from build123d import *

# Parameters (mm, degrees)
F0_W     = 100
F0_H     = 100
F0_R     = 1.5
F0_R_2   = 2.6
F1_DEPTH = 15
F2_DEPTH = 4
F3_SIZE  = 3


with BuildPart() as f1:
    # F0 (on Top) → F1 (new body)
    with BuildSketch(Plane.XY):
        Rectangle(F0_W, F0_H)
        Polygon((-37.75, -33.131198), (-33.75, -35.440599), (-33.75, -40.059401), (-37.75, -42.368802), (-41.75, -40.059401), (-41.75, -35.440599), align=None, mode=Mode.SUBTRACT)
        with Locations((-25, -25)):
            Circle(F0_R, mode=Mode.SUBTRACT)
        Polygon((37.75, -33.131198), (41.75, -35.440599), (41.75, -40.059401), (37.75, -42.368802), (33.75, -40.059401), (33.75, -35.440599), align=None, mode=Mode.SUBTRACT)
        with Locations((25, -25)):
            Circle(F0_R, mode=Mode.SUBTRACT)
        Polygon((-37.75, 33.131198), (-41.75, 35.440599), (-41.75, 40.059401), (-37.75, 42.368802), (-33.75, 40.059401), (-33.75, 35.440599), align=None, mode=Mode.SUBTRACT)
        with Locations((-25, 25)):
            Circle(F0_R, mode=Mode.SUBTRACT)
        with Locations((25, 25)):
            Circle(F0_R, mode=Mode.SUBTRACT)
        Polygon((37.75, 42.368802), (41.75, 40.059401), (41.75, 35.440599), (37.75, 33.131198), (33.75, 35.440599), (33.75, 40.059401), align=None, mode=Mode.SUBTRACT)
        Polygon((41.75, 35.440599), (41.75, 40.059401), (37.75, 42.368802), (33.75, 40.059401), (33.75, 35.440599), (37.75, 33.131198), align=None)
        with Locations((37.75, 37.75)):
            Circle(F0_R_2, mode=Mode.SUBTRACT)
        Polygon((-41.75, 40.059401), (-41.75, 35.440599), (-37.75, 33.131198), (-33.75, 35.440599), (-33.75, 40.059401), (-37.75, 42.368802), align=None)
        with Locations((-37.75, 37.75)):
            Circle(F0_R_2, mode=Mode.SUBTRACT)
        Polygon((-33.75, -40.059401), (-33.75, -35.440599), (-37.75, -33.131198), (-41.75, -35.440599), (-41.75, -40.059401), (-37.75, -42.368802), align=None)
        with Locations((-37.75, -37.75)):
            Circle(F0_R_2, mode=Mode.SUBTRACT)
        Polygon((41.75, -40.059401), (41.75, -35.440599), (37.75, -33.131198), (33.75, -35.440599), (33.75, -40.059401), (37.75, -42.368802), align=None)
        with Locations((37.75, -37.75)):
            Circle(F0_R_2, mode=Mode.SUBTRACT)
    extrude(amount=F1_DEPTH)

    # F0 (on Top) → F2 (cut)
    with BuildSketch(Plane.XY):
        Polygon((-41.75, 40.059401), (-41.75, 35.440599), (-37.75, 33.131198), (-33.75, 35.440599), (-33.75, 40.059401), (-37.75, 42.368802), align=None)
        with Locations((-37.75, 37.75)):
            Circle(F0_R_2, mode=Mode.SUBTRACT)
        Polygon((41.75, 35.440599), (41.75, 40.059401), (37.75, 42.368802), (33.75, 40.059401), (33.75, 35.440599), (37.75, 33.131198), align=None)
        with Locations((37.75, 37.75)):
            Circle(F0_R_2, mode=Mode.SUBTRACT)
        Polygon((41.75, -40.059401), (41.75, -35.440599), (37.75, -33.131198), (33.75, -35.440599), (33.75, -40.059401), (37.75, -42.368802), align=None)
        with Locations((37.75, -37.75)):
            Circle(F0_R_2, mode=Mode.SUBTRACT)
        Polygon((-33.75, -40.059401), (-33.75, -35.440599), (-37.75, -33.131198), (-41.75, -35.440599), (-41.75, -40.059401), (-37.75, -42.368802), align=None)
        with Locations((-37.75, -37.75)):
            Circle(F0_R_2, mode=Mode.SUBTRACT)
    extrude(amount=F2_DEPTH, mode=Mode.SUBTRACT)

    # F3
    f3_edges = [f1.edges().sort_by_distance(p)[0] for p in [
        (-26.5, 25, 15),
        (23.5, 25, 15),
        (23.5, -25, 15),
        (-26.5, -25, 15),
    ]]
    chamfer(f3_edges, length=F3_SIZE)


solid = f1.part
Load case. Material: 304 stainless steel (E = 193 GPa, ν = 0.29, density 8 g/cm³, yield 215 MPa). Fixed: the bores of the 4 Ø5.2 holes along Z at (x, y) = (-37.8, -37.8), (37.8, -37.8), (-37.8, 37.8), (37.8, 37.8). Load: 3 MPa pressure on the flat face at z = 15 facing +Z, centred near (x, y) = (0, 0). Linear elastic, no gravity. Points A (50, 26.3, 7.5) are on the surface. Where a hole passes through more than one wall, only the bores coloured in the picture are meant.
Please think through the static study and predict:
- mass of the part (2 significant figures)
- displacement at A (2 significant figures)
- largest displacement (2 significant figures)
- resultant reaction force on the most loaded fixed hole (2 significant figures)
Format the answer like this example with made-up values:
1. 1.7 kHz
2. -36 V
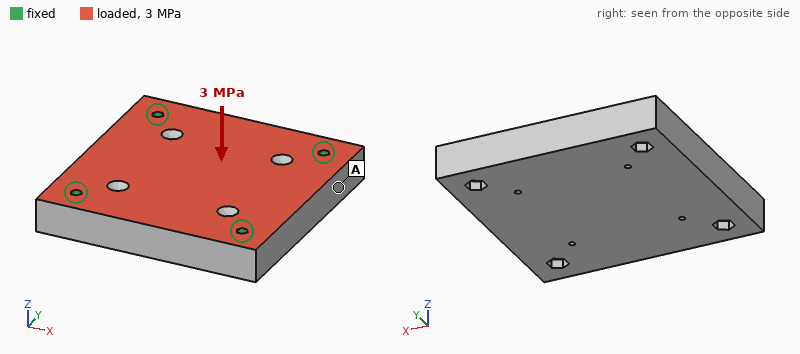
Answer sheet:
1. 1.2 kg
2. 3.2 µm
3. 21 µm
4. 7.4 kN
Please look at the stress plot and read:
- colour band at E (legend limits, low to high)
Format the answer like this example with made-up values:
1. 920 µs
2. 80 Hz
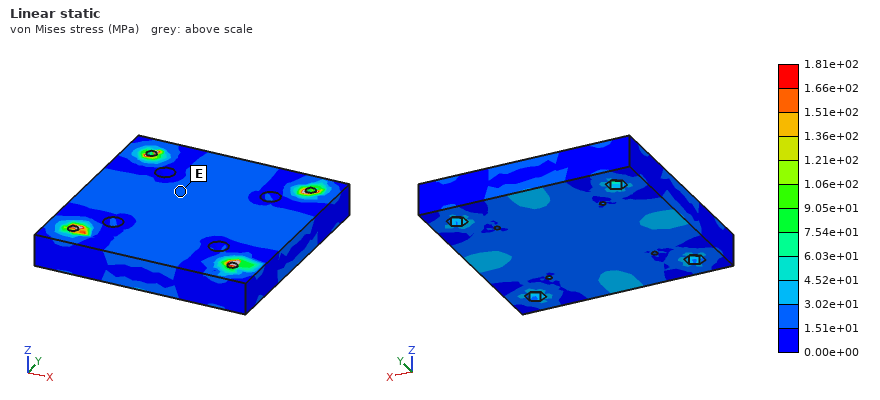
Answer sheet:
1. 1.51e+01 to 3.02e+01 MPa
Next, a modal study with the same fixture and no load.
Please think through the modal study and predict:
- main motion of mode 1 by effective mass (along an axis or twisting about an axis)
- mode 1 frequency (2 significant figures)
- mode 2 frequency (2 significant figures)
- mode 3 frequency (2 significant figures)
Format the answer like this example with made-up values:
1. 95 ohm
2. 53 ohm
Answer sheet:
1. along Z
2. 6400 Hz
3. 9800 Hz
4. 9800 Hz
